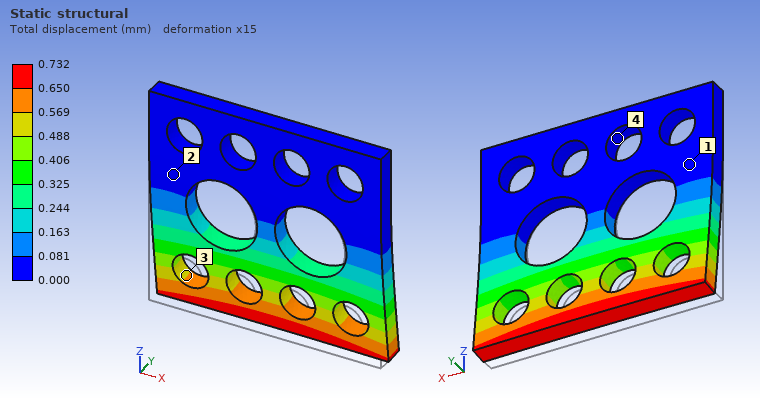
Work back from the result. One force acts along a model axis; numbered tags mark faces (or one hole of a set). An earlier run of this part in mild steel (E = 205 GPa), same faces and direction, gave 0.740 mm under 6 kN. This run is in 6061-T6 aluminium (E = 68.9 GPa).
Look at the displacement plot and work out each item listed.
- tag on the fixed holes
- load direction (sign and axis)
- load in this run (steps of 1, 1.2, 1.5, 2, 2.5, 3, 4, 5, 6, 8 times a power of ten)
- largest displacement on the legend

4
+Y
2 kN
0.732 mm
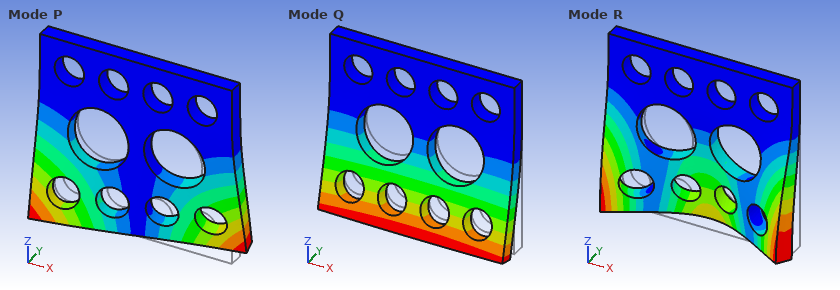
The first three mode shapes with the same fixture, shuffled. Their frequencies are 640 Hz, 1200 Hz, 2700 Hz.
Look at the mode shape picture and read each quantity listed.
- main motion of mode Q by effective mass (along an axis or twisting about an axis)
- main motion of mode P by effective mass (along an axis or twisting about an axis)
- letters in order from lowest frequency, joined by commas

along Y
twisting about Z
Q, P, R
